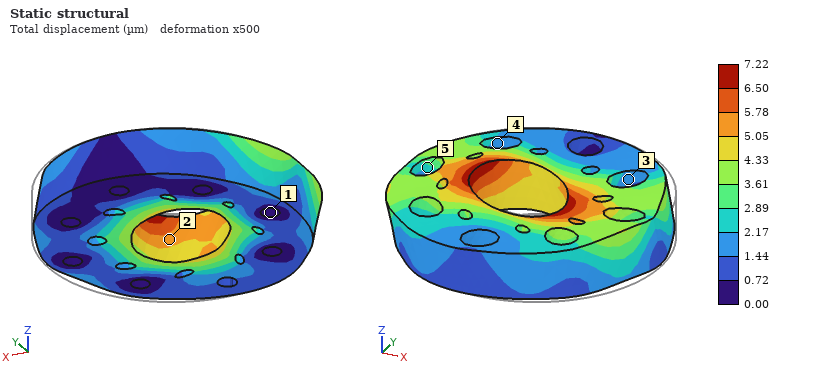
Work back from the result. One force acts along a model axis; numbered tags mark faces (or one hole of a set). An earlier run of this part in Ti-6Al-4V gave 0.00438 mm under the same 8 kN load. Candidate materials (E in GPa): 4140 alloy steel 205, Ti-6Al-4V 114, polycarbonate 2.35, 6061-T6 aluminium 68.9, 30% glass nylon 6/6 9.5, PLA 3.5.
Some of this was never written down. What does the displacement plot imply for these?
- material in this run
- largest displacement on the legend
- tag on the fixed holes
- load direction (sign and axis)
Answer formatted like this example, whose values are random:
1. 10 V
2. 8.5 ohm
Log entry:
1. 6061-T6 aluminium
2. 7.22 µm
3. 1
4. -X
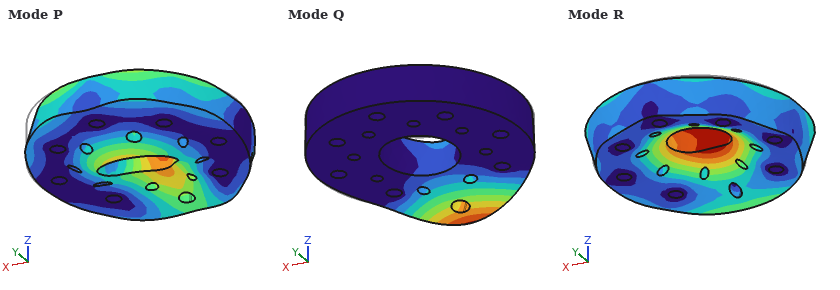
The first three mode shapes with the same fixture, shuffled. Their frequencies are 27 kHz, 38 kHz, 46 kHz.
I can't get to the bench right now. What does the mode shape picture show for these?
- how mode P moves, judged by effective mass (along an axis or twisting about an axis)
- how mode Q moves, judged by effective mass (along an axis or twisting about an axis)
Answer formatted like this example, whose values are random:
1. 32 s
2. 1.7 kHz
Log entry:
1. along Y
2. along Z
